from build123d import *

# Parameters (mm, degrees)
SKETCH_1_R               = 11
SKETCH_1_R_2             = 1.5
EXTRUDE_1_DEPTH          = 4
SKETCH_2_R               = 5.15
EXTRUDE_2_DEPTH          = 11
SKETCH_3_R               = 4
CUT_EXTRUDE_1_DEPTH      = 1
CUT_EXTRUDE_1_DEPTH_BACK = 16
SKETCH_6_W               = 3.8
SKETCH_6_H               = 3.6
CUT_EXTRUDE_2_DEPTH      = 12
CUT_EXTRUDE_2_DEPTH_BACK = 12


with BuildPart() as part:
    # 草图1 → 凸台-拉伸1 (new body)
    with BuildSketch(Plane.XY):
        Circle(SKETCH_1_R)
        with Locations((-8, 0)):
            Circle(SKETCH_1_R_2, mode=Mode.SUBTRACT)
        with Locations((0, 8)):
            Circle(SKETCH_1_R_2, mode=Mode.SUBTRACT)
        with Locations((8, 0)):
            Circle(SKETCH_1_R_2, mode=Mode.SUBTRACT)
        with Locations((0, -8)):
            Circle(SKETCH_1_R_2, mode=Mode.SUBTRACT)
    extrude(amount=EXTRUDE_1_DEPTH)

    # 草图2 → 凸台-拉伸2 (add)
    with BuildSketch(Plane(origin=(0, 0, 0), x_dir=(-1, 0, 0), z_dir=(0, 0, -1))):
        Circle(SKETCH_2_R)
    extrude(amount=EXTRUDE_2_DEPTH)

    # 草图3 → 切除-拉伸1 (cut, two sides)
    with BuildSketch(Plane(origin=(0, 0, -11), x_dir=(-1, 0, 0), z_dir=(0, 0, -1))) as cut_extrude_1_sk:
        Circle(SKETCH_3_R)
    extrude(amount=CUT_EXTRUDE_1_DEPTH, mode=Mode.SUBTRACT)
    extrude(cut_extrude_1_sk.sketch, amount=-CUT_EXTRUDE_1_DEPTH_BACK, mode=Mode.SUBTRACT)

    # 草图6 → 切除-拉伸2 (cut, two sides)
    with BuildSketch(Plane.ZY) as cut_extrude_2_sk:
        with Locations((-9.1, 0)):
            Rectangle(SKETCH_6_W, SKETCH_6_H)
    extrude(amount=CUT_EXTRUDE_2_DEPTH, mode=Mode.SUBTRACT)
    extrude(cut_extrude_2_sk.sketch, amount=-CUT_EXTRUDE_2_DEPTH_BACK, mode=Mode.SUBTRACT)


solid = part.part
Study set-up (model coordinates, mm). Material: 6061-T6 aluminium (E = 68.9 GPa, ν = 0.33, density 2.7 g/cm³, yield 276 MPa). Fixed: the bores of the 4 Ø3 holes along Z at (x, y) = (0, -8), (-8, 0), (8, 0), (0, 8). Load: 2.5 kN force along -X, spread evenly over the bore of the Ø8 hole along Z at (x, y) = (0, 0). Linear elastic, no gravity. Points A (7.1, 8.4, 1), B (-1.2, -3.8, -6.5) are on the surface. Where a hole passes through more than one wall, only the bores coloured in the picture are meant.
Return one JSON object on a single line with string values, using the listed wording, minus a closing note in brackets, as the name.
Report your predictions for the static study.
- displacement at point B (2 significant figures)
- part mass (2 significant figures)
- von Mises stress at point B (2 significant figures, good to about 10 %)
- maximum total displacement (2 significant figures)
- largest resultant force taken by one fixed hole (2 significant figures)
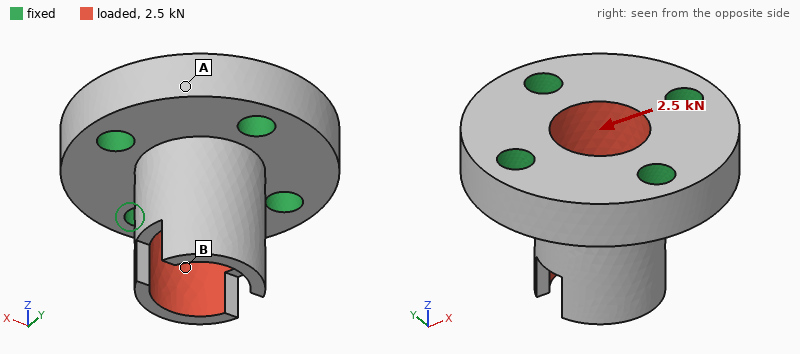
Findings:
{"displacement at point B": "34 µm", "part mass": "4.2 g", "von Mises stress at point B": "110 MPa", "maximum total displacement": "71 µm", "largest resultant force taken by one fixed hole": "1.1 kN"}
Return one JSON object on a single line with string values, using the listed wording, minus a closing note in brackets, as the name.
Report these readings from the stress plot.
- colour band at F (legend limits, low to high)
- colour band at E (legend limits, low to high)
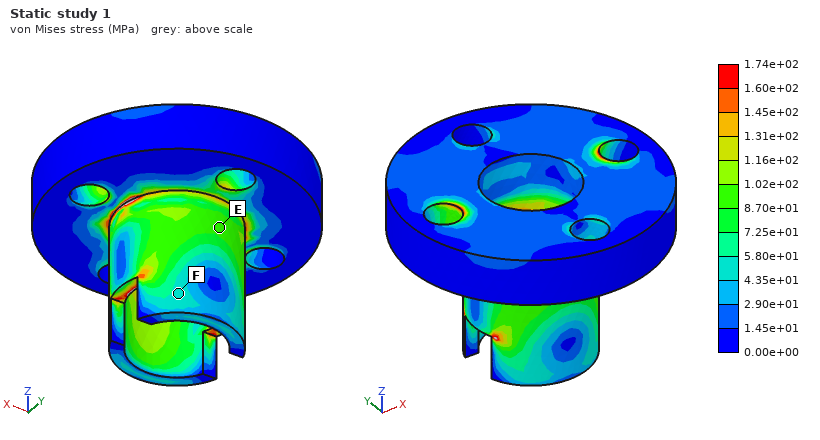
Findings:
{"colour band at F": "4.35e+01 to 5.80e+01 MPa", "colour band at E": "8.70e+01 to 1.02e+02 MPa"}
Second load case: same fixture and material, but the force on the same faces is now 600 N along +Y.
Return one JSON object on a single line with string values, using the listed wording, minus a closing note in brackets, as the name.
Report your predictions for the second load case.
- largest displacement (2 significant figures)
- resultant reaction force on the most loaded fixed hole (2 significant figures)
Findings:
{"largest displacement": "15 µm", "resultant reaction force on the most loaded fixed hole": "270 N"}
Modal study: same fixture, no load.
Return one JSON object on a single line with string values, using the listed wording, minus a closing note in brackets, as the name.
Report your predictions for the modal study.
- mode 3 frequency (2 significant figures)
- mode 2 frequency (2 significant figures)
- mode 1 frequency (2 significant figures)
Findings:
{"mode 3 frequency": "35 kHz", "mode 2 frequency": "35 kHz", "mode 1 frequency": "31 kHz"}
